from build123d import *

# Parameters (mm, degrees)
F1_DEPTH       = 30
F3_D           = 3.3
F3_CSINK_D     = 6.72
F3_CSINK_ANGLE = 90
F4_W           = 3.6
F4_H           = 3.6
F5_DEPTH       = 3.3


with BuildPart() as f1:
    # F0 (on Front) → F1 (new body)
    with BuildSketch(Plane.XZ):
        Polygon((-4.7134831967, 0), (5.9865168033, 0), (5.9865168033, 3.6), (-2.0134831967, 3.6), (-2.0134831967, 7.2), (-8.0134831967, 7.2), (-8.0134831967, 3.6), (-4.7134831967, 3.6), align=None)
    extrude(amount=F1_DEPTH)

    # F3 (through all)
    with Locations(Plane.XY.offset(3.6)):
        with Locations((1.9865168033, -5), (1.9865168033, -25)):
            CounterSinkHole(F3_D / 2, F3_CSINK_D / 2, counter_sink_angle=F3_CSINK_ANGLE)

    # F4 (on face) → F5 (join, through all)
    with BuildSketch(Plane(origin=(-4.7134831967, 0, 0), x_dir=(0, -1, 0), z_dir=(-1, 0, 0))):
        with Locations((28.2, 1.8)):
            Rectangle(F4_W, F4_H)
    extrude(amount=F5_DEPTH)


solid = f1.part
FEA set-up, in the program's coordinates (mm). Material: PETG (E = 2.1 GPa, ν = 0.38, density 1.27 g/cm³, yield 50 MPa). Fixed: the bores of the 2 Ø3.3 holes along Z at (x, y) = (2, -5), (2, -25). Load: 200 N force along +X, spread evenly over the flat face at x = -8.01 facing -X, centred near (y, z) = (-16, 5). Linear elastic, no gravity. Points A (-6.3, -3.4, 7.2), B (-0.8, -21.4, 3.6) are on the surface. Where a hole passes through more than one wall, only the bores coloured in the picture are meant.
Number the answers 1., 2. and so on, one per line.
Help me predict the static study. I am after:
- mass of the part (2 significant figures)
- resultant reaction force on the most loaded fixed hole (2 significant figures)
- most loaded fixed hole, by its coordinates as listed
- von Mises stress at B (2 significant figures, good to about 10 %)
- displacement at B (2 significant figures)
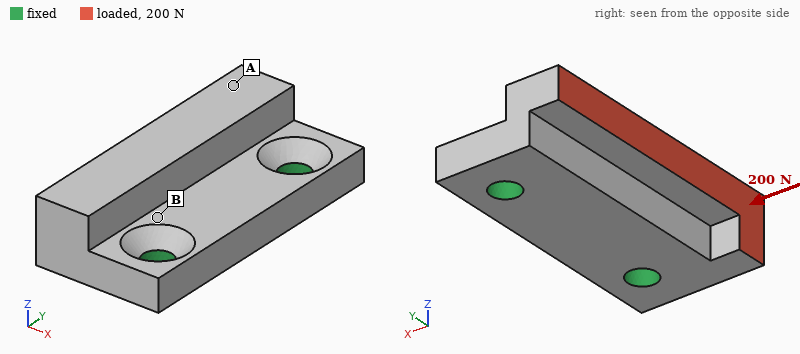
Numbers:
1. 2.2 g
2. 110 N
3. (2, -25)
4. 12 MPa
5. 0.083 mm
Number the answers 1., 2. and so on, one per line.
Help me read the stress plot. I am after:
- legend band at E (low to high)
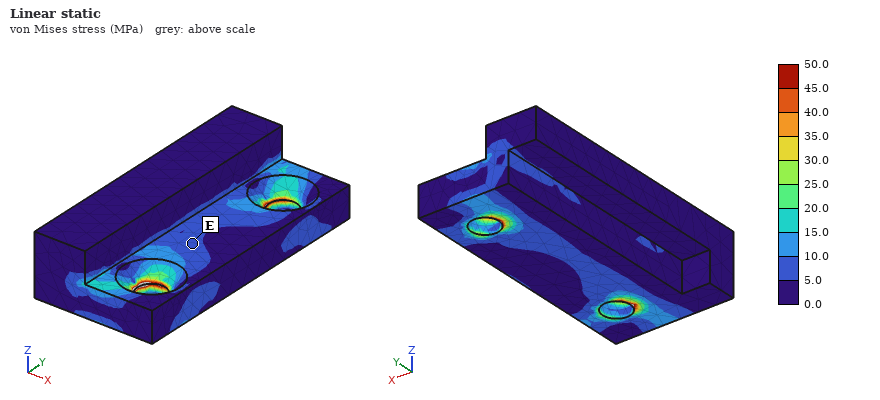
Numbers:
1. 5.0 to 10.0 MPa
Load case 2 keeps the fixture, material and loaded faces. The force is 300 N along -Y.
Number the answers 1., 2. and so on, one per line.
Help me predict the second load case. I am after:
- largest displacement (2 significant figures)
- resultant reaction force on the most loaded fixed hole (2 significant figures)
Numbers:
1. 0.14 mm
2. 210 N
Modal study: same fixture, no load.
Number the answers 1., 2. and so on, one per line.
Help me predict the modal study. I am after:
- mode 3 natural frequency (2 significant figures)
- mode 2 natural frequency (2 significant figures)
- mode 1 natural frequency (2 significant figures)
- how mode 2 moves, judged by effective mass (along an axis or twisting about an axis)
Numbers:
1. 8700 Hz
2. 5400 Hz
3. 3400 Hz
4. twisting about X
